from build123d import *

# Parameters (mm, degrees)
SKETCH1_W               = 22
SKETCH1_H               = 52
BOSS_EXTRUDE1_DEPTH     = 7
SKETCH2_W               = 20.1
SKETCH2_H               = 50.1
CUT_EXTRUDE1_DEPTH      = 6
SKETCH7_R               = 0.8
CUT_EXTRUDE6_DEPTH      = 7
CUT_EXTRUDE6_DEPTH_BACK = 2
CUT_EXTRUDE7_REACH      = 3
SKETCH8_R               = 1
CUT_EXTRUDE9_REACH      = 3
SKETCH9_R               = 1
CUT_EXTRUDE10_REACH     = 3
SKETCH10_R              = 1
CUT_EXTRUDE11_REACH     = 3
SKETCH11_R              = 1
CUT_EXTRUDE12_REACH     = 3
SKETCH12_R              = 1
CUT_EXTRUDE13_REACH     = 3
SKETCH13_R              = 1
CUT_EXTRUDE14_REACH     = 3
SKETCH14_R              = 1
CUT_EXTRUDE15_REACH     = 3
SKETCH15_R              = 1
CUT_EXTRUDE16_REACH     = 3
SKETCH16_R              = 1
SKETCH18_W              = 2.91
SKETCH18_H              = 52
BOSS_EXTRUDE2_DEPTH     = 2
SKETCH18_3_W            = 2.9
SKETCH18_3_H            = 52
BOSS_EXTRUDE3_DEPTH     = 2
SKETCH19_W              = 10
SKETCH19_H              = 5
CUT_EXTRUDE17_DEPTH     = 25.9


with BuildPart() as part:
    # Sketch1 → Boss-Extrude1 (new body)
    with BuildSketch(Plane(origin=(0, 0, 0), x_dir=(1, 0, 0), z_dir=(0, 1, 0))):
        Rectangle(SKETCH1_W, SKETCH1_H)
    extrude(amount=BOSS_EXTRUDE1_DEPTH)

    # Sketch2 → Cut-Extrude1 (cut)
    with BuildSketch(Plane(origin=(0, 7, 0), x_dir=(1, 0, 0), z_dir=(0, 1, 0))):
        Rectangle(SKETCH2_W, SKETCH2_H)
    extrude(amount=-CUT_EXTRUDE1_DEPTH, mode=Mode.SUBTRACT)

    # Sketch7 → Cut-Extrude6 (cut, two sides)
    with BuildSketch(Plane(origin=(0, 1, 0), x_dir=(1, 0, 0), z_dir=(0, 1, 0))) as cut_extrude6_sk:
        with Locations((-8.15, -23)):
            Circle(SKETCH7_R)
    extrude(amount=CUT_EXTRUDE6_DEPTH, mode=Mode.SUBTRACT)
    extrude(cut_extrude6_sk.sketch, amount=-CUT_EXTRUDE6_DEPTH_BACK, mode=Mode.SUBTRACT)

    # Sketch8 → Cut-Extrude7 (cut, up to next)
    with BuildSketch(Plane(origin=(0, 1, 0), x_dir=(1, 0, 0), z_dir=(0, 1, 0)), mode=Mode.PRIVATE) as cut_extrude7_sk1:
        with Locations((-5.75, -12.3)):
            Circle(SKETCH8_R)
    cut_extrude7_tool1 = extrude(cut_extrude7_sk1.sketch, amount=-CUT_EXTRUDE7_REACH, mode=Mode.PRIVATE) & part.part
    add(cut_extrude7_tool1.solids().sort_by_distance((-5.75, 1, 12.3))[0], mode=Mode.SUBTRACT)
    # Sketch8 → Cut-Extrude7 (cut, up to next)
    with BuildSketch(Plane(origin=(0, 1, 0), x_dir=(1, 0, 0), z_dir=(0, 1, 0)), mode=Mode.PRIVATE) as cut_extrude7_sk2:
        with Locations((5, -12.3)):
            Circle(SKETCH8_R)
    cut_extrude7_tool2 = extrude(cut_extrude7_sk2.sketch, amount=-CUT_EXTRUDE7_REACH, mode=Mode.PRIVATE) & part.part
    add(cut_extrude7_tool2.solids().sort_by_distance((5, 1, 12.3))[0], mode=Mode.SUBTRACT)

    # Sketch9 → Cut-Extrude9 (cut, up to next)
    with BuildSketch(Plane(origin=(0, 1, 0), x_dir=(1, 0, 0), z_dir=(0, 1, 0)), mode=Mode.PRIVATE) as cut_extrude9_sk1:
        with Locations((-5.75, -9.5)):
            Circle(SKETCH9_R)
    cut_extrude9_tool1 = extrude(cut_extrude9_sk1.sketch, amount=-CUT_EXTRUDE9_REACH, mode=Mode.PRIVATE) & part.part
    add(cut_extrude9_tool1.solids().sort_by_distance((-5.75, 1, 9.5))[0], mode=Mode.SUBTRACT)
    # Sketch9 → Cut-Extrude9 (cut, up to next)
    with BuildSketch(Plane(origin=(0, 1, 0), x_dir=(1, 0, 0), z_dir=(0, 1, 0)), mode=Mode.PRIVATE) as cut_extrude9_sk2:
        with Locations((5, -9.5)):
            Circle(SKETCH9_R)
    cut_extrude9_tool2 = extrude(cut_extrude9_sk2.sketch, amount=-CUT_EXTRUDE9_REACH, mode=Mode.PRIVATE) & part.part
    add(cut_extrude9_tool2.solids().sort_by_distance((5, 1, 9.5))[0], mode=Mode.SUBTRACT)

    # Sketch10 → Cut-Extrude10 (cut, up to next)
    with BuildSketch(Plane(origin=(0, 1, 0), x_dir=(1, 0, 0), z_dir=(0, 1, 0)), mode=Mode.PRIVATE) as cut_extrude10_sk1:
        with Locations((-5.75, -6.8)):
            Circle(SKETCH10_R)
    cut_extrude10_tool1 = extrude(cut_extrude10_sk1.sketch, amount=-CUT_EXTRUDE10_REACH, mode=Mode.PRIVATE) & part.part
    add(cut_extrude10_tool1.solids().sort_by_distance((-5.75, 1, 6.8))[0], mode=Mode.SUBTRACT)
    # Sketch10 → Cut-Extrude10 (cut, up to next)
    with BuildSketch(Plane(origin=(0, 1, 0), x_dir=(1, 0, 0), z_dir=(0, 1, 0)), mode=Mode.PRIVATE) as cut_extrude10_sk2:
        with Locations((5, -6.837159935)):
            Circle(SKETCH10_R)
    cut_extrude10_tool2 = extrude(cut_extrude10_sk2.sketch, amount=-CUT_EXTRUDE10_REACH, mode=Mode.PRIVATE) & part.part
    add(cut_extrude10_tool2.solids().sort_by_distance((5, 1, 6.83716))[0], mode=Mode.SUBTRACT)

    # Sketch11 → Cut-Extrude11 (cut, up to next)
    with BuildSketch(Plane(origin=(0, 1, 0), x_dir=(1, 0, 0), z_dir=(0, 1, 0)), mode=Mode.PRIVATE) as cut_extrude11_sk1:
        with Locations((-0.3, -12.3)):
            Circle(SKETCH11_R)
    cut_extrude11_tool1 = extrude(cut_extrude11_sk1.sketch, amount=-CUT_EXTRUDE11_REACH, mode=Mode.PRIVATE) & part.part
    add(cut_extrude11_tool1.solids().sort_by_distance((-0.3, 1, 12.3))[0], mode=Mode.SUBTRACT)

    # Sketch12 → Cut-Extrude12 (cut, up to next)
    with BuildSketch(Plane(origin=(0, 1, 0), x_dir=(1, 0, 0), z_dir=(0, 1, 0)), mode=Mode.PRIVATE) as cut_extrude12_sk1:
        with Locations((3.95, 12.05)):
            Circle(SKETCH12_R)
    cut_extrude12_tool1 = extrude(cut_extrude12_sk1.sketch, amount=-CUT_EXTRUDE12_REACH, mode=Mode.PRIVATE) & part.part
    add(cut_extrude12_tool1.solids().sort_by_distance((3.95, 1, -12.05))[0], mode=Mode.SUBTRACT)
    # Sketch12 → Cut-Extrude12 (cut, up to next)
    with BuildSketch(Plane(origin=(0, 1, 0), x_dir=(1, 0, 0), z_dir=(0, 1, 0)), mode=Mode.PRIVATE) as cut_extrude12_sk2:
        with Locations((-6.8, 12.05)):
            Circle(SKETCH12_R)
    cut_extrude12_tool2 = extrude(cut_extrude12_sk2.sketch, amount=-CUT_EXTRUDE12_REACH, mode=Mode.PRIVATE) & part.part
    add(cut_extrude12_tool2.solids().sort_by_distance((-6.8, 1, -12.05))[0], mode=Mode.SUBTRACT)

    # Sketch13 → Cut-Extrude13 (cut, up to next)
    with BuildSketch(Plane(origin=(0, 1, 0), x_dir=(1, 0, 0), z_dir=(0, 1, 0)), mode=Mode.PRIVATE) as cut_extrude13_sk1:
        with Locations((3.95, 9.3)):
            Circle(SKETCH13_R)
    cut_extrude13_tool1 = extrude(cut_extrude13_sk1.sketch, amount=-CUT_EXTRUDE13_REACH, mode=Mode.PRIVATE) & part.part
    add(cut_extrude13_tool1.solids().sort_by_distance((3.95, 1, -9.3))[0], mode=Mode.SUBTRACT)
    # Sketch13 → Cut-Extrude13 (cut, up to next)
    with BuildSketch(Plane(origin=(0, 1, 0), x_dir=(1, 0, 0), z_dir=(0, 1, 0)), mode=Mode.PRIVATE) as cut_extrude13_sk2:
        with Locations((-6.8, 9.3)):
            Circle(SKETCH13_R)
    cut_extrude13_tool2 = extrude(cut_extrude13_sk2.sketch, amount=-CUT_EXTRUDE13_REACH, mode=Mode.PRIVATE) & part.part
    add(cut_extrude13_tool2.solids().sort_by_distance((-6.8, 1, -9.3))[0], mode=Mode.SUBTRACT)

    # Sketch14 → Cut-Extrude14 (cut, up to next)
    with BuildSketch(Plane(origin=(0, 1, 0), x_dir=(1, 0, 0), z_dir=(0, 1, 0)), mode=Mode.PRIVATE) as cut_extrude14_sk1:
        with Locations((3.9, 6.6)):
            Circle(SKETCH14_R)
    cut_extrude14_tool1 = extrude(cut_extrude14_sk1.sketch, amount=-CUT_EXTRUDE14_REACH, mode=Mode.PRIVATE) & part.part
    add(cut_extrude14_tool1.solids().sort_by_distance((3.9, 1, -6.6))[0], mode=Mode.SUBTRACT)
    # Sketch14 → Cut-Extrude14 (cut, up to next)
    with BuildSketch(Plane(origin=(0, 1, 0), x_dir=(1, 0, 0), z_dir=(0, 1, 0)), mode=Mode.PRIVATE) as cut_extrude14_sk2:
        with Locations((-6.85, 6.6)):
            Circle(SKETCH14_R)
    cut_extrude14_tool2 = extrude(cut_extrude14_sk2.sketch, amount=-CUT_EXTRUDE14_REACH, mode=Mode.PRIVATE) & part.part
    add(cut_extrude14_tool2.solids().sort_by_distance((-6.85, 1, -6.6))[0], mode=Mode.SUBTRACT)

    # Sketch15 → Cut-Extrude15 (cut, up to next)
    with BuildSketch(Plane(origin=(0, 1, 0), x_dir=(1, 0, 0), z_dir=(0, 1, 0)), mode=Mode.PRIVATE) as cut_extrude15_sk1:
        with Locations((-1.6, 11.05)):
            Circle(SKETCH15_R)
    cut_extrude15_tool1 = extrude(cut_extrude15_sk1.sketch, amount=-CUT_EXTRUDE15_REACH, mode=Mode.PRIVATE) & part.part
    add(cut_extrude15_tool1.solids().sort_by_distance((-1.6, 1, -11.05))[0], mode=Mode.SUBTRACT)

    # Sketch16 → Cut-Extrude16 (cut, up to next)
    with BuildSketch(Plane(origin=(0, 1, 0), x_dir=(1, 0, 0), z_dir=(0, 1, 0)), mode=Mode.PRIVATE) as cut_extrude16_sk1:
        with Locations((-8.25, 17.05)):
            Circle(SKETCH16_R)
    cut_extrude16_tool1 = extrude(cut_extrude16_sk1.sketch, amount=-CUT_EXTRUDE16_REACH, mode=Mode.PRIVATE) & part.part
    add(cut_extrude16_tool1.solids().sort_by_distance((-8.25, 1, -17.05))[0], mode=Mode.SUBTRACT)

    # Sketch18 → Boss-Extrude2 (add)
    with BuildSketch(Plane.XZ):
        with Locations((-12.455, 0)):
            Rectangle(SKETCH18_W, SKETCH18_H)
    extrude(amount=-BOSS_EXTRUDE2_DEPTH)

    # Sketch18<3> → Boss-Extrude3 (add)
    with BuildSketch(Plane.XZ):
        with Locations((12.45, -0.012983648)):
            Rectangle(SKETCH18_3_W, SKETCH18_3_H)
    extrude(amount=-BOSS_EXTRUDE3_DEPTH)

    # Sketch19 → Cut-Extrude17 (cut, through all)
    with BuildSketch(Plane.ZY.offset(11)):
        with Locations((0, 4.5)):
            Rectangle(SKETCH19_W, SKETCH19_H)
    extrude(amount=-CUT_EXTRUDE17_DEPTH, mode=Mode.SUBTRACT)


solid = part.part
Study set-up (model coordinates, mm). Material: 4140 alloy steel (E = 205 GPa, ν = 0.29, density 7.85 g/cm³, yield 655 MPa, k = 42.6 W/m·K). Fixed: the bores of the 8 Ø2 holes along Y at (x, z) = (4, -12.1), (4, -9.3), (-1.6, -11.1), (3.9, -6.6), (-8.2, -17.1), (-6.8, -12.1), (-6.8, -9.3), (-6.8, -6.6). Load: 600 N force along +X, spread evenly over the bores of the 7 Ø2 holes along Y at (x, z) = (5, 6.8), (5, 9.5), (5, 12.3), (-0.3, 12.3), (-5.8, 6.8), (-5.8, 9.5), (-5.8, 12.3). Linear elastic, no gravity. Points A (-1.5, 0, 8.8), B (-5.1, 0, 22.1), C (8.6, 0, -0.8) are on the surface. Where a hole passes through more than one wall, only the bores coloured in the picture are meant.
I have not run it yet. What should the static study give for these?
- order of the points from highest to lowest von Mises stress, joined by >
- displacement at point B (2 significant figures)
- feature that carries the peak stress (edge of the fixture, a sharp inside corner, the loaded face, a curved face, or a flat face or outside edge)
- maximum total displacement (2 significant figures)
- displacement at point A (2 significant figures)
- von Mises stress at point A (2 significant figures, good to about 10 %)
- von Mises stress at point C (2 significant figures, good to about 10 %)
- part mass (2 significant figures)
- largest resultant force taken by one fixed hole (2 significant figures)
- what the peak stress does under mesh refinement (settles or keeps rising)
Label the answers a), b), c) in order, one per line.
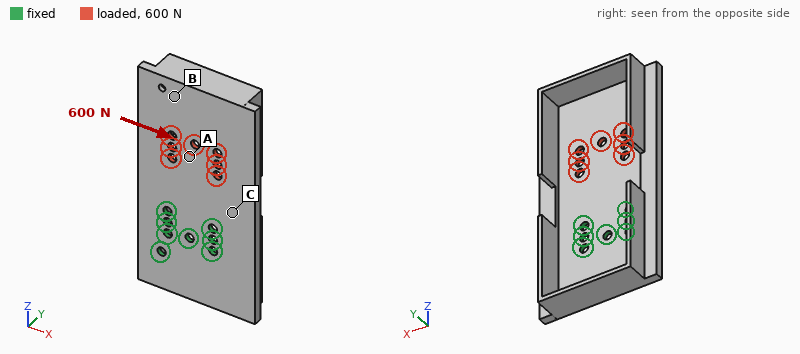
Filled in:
a) A > C > B
b) 18 µm
c) edge of the fixture
d) 28 µm
e) 10 µm
f) 39 MPa
g) 27 MPa
h) 19 g
i) 500 N
j) keeps rising
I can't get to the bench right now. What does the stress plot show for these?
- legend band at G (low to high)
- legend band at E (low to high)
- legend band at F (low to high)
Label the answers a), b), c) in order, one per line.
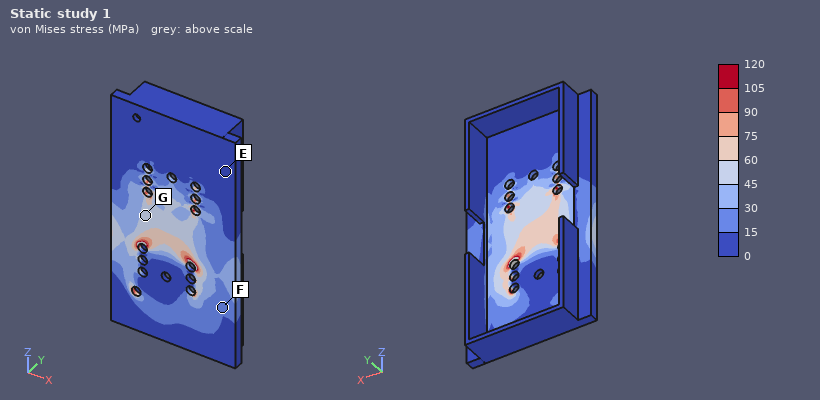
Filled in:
a) 45 to 60 MPa
b) 0 to 15 MPa
c) 15 to 30 MPa
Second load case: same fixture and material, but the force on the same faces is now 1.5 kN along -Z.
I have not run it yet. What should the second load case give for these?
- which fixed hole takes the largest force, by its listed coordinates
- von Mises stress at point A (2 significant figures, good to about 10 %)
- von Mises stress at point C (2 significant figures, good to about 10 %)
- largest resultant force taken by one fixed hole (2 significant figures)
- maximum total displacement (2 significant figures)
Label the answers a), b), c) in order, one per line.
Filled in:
a) (3.9, -6.6)
b) 55 MPa
c) 54 MPa
d) 490 N
e) 46 µm
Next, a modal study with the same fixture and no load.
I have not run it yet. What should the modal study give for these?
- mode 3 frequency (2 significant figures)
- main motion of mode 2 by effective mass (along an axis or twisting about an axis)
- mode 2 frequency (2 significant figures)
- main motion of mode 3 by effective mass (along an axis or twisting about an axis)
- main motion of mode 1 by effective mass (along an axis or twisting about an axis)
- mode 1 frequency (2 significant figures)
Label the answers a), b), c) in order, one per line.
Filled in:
a) 4400 Hz
b) twisting about Z
c) 2100 Hz
d) along Y
e) along Y
f) 990 Hz
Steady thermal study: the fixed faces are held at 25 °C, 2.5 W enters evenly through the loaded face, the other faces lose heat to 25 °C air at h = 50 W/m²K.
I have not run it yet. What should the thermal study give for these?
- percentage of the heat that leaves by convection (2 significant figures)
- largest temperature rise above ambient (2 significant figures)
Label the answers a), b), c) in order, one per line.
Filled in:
a) 57 %
b) 19 K
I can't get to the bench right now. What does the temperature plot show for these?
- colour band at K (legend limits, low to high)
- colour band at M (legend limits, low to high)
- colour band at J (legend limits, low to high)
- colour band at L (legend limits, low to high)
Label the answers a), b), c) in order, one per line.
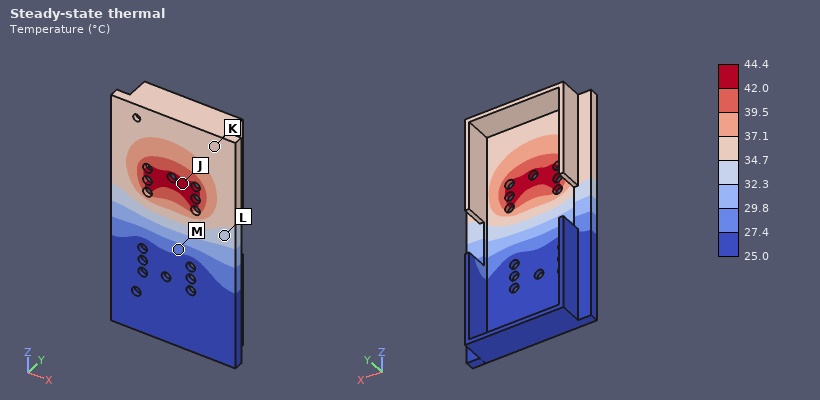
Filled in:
a) 34.7 to 37.1 °C
b) 27.4 to 29.8 °C
c) 42.0 to 44.4 °C
d) 32.3 to 34.7 °C
